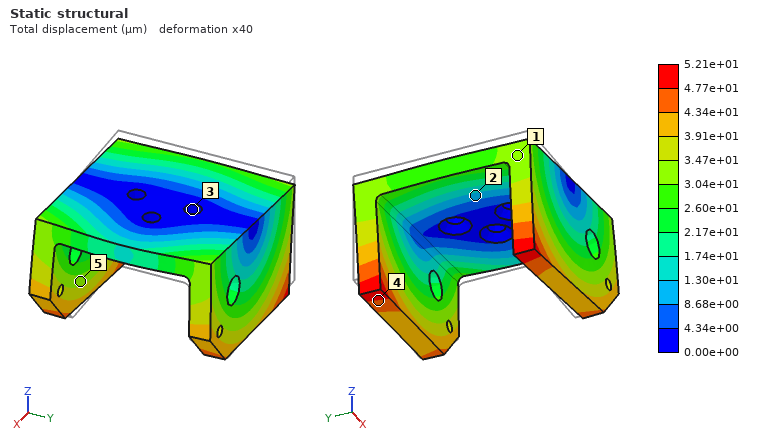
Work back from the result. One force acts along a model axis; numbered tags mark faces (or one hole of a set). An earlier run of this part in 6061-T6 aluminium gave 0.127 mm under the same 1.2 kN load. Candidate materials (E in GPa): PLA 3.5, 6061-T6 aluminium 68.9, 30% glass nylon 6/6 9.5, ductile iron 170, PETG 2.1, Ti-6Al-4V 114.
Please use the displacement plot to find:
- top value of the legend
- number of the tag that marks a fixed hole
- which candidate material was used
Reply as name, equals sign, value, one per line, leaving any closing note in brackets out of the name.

top value of the legend = 5.21e+01 µm
number of the tag that marks a fixed hole = 3
which candidate material was used = ductile iron
